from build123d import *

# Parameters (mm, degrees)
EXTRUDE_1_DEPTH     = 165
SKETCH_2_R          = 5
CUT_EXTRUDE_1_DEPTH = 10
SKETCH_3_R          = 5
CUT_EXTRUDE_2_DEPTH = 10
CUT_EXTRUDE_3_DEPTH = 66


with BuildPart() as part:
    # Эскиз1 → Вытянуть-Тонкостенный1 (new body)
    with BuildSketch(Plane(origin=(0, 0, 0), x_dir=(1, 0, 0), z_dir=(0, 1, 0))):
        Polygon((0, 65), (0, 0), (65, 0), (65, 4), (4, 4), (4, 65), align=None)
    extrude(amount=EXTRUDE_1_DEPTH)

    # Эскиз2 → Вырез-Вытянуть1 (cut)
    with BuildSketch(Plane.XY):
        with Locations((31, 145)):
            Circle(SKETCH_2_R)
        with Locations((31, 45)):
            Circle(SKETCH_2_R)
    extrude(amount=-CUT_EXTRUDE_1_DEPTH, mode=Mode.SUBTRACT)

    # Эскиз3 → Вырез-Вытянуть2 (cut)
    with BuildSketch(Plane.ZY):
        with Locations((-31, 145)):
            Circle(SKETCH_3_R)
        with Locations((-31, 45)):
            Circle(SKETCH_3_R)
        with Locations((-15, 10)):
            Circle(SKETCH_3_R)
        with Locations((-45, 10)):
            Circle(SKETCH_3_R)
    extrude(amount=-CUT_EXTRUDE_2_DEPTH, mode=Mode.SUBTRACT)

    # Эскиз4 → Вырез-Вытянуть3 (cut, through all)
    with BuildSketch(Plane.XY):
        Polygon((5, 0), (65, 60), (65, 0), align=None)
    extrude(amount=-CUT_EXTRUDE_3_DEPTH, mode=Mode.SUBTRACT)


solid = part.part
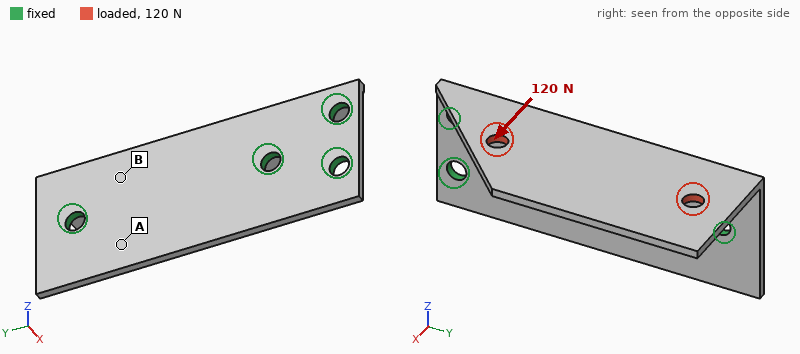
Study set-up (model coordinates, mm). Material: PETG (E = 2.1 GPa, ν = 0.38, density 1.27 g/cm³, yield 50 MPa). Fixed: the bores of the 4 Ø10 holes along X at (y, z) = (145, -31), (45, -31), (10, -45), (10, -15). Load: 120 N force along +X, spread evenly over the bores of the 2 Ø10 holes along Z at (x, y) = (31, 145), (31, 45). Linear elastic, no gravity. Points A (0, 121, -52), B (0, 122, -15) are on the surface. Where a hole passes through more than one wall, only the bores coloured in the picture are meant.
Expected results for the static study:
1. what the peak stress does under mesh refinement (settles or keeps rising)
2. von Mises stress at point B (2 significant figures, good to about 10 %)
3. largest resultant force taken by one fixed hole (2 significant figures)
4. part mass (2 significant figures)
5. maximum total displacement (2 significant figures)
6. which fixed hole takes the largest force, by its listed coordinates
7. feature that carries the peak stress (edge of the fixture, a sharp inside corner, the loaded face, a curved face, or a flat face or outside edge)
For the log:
keeps rising
3.0 MPa
70 N
94 g
2.0 mm
(145, -31)
edge of the fixture
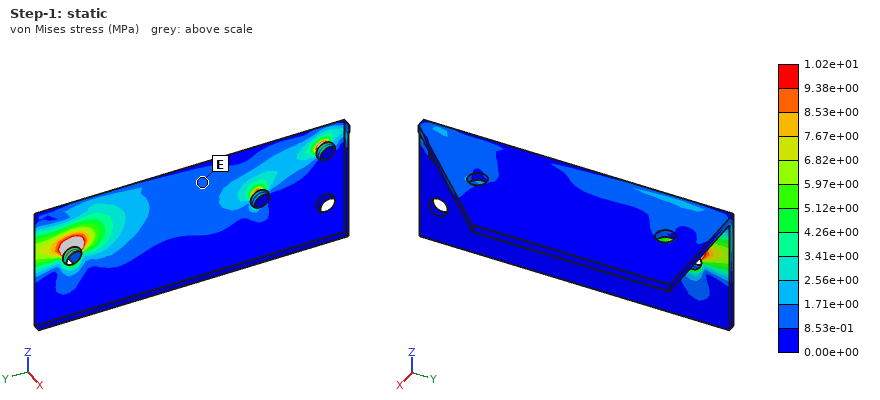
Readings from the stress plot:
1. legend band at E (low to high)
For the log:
8.53e-01 to 1.71e+00 MPa
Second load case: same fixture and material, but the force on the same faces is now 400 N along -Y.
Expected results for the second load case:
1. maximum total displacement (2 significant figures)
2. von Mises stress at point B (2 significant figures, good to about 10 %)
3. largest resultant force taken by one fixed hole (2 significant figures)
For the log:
2.3 mm
2.8 MPa
170 N
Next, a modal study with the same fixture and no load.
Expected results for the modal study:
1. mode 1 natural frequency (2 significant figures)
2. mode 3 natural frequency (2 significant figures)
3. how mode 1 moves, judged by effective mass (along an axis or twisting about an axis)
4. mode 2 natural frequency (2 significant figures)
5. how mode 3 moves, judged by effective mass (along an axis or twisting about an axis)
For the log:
140 Hz
420 Hz
along Z
320 Hz
along X
